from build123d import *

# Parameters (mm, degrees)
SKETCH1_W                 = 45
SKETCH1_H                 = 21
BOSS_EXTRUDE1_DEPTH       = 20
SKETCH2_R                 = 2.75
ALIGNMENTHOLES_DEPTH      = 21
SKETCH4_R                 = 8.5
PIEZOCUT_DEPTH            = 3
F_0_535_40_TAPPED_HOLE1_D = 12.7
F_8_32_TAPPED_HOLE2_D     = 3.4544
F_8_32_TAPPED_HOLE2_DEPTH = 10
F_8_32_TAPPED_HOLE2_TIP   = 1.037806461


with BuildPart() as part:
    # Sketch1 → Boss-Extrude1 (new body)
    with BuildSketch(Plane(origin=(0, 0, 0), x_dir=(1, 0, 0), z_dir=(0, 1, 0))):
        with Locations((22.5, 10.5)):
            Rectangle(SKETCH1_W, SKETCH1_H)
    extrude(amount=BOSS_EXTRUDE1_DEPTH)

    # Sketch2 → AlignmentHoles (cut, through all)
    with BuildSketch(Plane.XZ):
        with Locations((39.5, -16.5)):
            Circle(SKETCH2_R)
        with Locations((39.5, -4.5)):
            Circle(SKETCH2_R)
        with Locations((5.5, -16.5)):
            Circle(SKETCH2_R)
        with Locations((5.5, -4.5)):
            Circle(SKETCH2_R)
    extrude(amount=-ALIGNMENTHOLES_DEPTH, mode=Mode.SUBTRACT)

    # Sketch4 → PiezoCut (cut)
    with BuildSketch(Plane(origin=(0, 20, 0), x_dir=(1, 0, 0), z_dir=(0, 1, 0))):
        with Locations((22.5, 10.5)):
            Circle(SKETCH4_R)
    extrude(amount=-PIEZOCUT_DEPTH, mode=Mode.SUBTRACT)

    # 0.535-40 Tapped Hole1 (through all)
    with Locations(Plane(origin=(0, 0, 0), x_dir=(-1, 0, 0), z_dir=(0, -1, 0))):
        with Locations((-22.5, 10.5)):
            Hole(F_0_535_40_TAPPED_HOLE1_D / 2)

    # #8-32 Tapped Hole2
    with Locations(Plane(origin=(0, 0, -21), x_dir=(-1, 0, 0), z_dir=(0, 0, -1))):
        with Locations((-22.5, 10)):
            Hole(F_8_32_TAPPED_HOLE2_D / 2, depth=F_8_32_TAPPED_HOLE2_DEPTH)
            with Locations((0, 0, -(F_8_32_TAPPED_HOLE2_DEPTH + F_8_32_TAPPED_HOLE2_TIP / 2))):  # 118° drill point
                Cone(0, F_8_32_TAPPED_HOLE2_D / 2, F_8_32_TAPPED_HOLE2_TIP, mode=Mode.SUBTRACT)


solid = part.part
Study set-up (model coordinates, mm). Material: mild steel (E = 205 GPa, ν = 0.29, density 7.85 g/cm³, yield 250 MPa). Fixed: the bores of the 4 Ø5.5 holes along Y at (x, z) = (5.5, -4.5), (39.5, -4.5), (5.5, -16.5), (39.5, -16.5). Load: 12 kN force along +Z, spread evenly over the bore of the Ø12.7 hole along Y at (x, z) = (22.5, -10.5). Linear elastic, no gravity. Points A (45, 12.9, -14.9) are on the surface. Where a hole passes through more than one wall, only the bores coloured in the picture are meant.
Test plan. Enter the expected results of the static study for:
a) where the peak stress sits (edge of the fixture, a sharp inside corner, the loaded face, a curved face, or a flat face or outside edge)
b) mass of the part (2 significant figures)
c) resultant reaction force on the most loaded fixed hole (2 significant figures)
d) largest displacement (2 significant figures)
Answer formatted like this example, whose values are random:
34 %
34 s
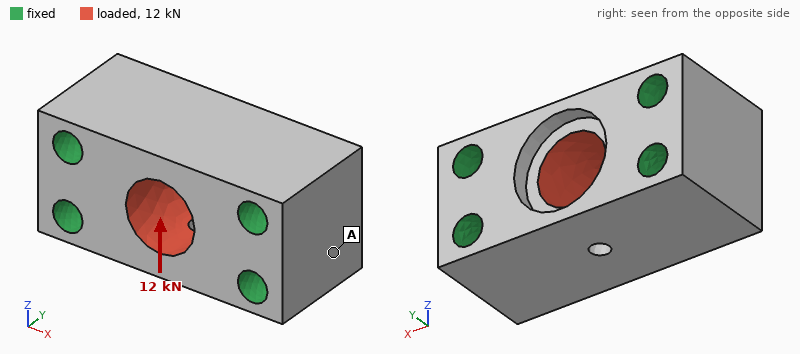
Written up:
a curved face
110 g
3.9 kN
4.9 µm
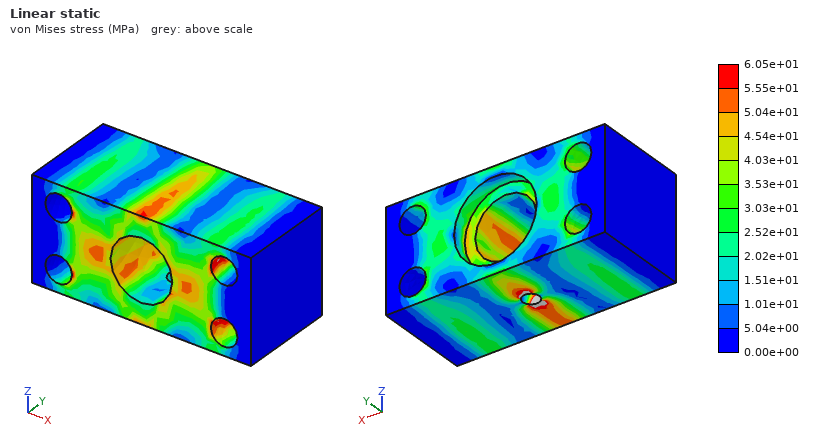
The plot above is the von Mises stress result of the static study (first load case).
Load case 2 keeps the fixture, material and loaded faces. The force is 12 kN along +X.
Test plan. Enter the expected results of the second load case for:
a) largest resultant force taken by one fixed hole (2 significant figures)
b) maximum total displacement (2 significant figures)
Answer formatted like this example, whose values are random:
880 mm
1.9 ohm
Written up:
3.1 kN
1.3 µm
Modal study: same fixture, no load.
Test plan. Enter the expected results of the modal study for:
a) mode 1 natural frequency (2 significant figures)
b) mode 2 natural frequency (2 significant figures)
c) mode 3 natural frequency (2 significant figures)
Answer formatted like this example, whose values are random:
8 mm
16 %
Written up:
52 kHz
53 kHz
54 kHz
